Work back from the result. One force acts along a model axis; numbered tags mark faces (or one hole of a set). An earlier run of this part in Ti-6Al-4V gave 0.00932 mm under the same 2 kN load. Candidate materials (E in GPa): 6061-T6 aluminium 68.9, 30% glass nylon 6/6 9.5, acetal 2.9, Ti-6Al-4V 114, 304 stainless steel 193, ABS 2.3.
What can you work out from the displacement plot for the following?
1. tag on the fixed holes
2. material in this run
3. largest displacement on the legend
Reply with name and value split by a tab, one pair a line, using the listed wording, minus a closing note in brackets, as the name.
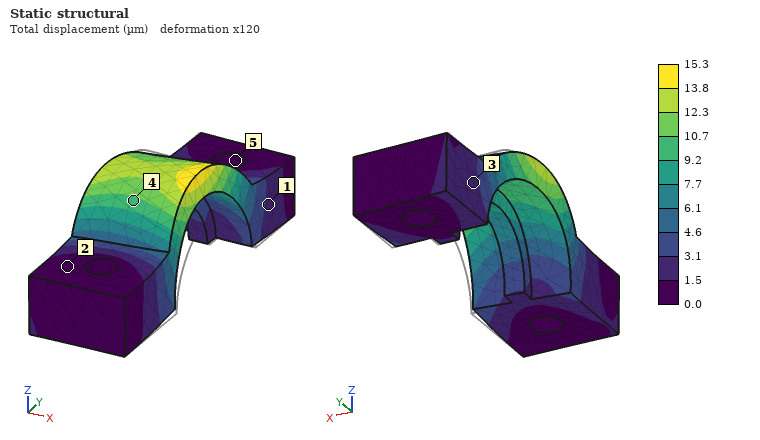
tag on the fixed holes	5
material in this run	6061-T6 aluminium
largest displacement on the legend	15.3 µm
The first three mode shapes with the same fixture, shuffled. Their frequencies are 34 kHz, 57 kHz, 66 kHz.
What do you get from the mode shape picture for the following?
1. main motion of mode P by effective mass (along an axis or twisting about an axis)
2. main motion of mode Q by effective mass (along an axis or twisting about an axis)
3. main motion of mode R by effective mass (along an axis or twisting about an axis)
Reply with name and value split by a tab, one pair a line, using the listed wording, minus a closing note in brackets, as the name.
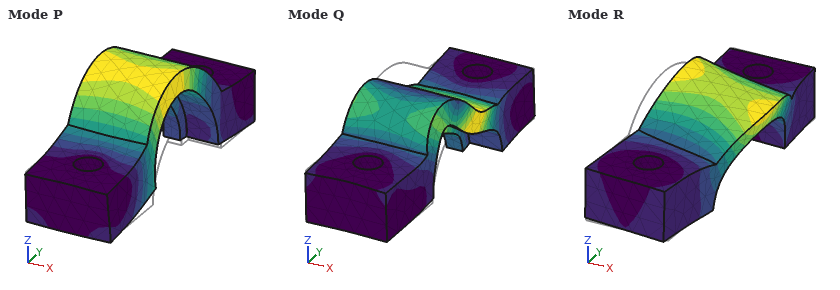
main motion of mode P by effective mass	along Z
main motion of mode Q by effective mass	along Y
main motion of mode R by effective mass	along X
